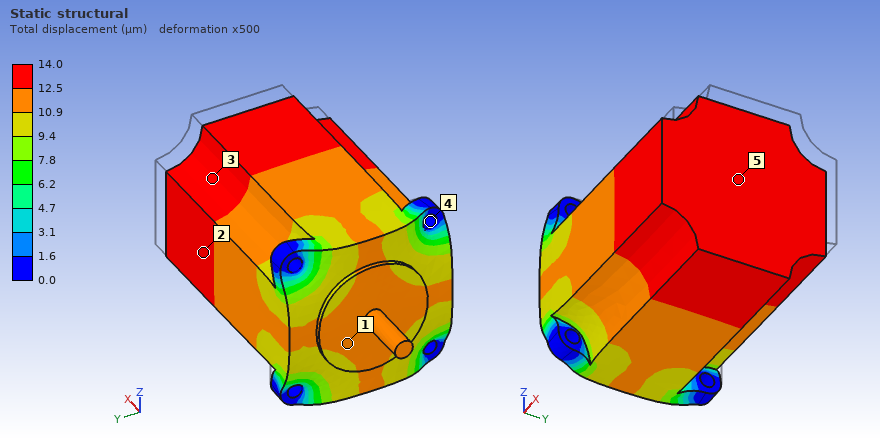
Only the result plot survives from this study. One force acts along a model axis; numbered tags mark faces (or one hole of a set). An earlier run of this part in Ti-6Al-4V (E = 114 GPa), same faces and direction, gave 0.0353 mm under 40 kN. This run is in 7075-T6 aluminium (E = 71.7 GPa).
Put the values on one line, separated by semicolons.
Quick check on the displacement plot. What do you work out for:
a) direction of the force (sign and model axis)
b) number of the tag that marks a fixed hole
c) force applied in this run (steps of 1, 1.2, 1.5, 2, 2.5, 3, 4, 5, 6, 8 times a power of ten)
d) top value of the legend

-X; 4; 10 kN; 14.0 µm
